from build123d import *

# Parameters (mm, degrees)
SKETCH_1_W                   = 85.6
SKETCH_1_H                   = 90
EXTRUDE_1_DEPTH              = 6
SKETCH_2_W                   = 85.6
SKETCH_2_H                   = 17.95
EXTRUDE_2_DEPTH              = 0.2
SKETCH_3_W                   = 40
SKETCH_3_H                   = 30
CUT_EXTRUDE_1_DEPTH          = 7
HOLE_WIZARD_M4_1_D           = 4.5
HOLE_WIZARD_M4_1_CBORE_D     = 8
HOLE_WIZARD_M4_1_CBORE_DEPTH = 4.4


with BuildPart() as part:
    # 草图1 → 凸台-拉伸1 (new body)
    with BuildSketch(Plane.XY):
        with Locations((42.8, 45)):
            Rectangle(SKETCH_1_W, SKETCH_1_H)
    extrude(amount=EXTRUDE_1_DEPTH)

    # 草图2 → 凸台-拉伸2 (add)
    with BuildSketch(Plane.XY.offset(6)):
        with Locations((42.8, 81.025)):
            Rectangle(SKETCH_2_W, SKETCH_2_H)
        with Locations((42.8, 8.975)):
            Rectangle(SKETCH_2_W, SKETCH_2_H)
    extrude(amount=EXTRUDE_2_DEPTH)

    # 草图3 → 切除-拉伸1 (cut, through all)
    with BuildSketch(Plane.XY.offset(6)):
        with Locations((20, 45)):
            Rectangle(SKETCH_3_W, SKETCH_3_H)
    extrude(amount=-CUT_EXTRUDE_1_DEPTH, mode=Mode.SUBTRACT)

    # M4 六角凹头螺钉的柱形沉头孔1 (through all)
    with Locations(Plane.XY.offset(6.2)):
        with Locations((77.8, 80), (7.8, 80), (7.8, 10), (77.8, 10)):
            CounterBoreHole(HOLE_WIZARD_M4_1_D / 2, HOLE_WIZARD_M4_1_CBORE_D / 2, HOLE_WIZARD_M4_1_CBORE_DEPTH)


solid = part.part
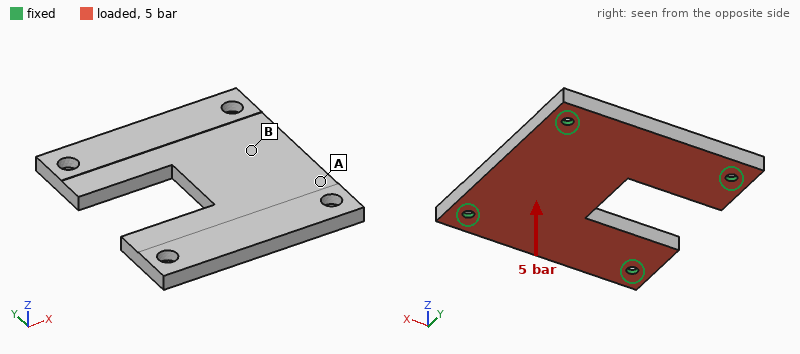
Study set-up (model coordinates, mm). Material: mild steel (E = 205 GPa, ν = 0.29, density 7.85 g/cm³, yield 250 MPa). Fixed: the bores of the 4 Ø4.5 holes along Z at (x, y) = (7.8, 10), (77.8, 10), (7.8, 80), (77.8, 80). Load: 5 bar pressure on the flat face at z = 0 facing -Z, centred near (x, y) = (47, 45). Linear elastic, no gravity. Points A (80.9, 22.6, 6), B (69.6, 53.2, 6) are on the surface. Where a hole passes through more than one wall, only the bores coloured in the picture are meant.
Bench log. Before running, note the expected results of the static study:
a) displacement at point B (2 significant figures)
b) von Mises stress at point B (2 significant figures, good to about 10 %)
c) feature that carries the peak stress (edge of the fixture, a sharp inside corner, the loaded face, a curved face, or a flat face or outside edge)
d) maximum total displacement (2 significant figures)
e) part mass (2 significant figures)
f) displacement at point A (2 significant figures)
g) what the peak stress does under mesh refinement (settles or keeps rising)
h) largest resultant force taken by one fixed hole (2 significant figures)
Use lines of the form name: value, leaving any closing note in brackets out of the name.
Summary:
displacement at point B: 25 µm
von Mises stress at point B: 29 MPa
feature that carries the peak stress: edge of the fixture
maximum total displacement: 44 µm
part mass: 300 g
displacement at point A: 9.4 µm
what the peak stress does under mesh refinement: keeps rising
largest resultant force taken by one fixed hole: 1.6 kN
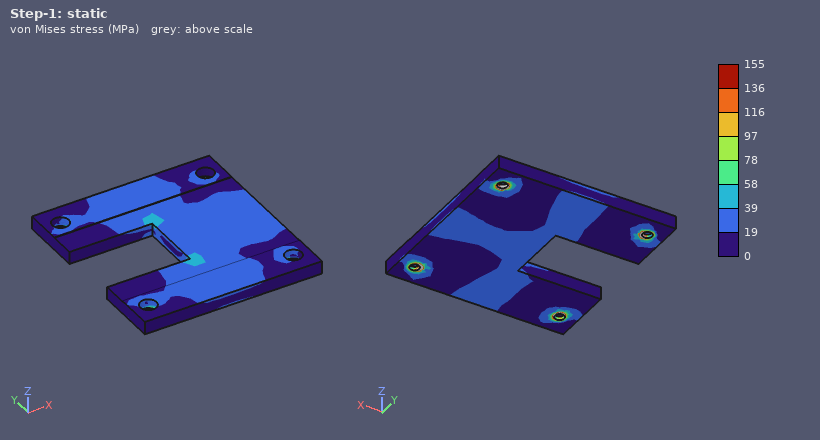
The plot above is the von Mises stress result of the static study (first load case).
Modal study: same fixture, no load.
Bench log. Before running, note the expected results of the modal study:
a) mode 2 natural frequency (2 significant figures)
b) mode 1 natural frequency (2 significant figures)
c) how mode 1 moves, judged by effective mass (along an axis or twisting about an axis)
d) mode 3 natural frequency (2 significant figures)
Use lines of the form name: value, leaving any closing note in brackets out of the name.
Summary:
mode 2 natural frequency: 5000 Hz
mode 1 natural frequency: 3200 Hz
how mode 1 moves, judged by effective mass: along Z
mode 3 natural frequency: 5100 Hz
